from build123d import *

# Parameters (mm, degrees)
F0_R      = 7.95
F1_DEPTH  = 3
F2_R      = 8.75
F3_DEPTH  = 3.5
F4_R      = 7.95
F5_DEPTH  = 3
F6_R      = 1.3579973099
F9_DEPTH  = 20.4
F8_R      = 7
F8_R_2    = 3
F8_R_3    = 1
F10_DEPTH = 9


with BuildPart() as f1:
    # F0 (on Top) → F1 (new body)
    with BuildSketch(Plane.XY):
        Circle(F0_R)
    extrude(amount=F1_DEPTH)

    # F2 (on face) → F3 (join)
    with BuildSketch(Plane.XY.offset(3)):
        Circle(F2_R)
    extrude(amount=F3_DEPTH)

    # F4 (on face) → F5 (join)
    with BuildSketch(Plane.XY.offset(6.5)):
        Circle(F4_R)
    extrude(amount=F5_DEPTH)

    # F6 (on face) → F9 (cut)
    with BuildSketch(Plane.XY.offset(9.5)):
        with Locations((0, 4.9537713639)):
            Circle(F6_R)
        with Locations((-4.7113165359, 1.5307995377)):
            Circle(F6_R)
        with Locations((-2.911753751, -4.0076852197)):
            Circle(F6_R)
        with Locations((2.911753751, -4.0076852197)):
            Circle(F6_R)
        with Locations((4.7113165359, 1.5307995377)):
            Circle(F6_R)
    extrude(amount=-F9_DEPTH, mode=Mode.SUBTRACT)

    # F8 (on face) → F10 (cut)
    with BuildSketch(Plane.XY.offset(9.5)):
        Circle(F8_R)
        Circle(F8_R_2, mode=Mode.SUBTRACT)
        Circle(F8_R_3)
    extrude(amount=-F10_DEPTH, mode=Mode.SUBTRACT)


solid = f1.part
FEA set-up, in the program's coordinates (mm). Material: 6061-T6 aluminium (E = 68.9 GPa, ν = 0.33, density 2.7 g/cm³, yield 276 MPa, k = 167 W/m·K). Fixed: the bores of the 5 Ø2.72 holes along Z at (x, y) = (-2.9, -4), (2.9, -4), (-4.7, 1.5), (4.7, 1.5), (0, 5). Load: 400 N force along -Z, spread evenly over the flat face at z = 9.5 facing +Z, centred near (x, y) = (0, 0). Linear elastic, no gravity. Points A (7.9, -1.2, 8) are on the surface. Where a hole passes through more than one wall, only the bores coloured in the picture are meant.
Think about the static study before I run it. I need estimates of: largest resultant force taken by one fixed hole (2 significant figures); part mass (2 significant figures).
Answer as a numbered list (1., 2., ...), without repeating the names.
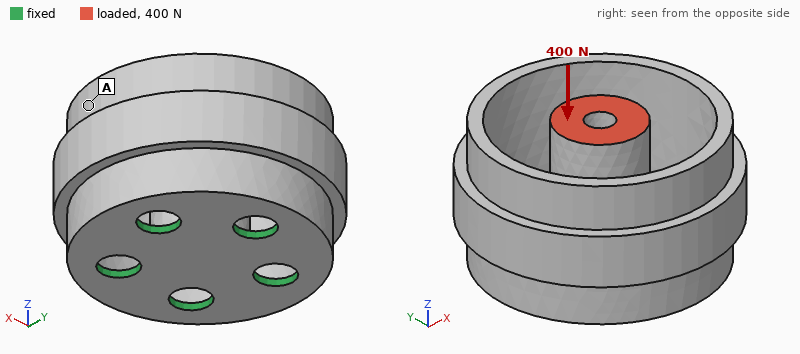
1. 93 N
2. 2.3 g
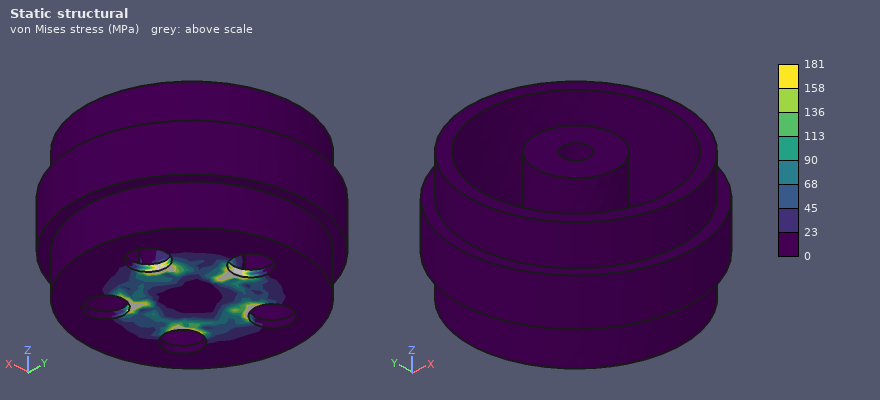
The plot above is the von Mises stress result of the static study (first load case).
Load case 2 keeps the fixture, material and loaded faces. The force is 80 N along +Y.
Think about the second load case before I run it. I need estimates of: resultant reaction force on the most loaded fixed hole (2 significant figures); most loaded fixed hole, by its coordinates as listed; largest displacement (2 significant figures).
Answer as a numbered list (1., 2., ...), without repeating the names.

1. 91 N
2. (0, 5)
3. 22 µm
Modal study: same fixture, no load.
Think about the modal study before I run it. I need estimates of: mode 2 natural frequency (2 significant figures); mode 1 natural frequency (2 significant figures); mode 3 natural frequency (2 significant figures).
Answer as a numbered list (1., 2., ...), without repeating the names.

1. 19 kHz
2. 19 kHz
3. 19 kHz
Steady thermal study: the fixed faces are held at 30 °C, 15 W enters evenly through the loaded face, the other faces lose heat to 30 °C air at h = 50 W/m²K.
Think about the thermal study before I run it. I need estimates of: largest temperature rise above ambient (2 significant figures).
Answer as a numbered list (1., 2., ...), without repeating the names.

1. 44 K
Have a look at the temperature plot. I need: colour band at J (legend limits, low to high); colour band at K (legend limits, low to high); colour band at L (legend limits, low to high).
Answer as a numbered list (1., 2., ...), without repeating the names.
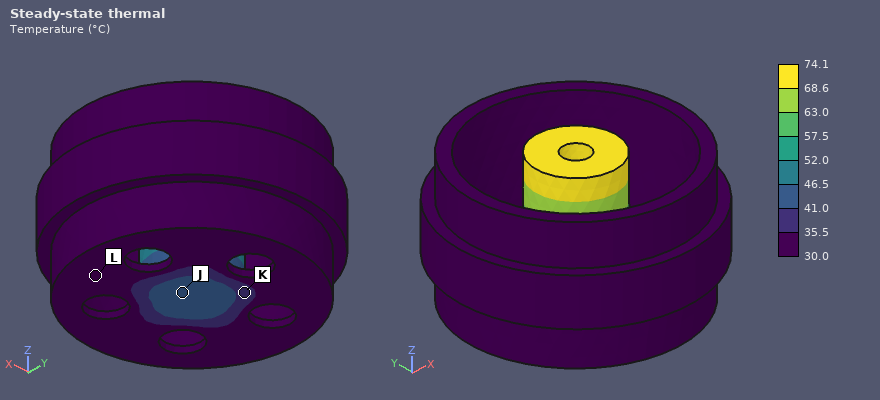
1. 41.0 to 46.5 °C
2. 35.5 to 41.0 °C
3. 30.0 to 35.5 °C
